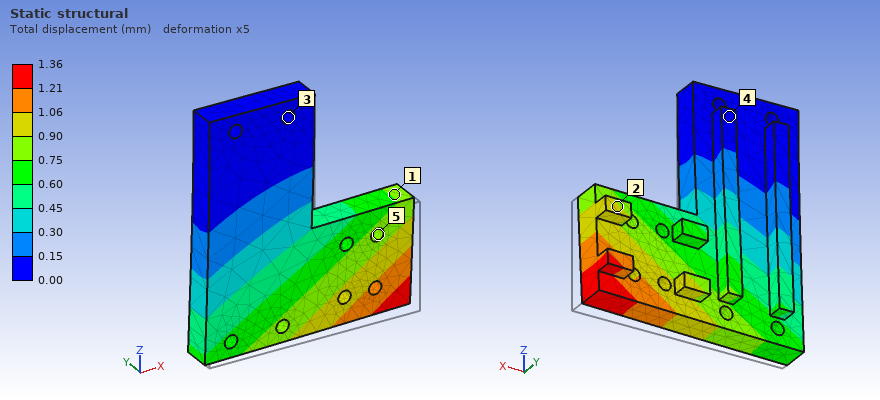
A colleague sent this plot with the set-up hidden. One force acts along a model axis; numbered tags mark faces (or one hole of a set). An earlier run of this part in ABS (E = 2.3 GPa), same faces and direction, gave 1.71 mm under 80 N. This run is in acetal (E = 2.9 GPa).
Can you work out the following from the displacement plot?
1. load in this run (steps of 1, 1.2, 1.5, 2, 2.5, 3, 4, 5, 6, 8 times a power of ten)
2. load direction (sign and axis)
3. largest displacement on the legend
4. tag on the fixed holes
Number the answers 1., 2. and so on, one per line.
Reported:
1. 80 N
2. +Y
3. 1.36 mm
4. 3
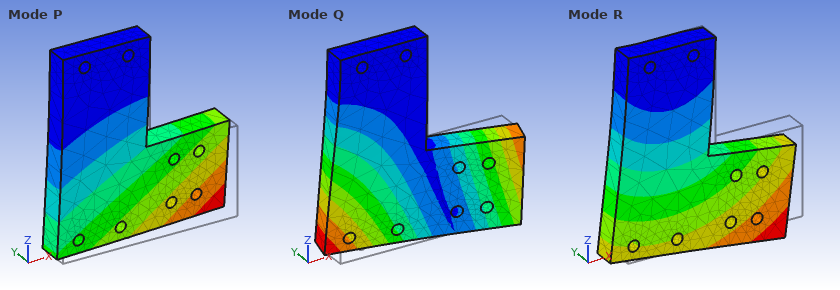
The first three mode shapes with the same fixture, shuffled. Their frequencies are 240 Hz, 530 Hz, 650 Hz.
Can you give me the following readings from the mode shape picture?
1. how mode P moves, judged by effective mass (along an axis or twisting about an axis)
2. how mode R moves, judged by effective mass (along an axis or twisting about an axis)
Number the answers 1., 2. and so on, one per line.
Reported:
1. along Y
2. along X
